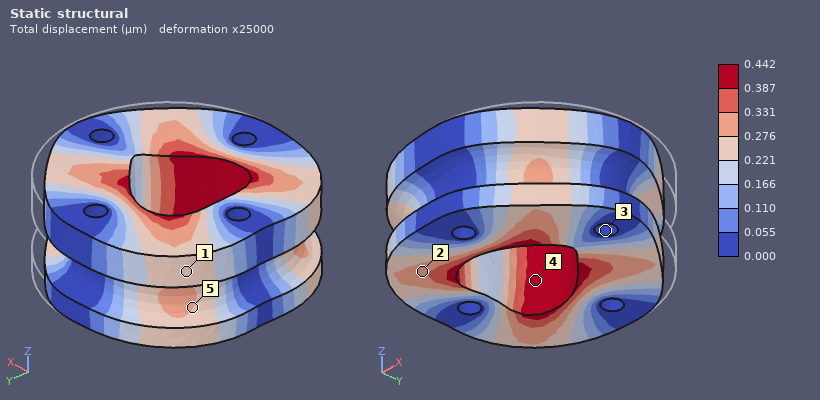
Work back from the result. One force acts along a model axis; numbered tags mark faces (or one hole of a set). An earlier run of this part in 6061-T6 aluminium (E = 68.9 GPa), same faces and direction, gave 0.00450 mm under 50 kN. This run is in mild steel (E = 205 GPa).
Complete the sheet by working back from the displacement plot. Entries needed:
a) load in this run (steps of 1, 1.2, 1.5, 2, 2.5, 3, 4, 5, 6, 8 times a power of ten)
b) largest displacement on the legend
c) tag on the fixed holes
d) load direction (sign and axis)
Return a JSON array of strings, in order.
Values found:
["15 kN", "0.442 µm", "3", "-X"]
